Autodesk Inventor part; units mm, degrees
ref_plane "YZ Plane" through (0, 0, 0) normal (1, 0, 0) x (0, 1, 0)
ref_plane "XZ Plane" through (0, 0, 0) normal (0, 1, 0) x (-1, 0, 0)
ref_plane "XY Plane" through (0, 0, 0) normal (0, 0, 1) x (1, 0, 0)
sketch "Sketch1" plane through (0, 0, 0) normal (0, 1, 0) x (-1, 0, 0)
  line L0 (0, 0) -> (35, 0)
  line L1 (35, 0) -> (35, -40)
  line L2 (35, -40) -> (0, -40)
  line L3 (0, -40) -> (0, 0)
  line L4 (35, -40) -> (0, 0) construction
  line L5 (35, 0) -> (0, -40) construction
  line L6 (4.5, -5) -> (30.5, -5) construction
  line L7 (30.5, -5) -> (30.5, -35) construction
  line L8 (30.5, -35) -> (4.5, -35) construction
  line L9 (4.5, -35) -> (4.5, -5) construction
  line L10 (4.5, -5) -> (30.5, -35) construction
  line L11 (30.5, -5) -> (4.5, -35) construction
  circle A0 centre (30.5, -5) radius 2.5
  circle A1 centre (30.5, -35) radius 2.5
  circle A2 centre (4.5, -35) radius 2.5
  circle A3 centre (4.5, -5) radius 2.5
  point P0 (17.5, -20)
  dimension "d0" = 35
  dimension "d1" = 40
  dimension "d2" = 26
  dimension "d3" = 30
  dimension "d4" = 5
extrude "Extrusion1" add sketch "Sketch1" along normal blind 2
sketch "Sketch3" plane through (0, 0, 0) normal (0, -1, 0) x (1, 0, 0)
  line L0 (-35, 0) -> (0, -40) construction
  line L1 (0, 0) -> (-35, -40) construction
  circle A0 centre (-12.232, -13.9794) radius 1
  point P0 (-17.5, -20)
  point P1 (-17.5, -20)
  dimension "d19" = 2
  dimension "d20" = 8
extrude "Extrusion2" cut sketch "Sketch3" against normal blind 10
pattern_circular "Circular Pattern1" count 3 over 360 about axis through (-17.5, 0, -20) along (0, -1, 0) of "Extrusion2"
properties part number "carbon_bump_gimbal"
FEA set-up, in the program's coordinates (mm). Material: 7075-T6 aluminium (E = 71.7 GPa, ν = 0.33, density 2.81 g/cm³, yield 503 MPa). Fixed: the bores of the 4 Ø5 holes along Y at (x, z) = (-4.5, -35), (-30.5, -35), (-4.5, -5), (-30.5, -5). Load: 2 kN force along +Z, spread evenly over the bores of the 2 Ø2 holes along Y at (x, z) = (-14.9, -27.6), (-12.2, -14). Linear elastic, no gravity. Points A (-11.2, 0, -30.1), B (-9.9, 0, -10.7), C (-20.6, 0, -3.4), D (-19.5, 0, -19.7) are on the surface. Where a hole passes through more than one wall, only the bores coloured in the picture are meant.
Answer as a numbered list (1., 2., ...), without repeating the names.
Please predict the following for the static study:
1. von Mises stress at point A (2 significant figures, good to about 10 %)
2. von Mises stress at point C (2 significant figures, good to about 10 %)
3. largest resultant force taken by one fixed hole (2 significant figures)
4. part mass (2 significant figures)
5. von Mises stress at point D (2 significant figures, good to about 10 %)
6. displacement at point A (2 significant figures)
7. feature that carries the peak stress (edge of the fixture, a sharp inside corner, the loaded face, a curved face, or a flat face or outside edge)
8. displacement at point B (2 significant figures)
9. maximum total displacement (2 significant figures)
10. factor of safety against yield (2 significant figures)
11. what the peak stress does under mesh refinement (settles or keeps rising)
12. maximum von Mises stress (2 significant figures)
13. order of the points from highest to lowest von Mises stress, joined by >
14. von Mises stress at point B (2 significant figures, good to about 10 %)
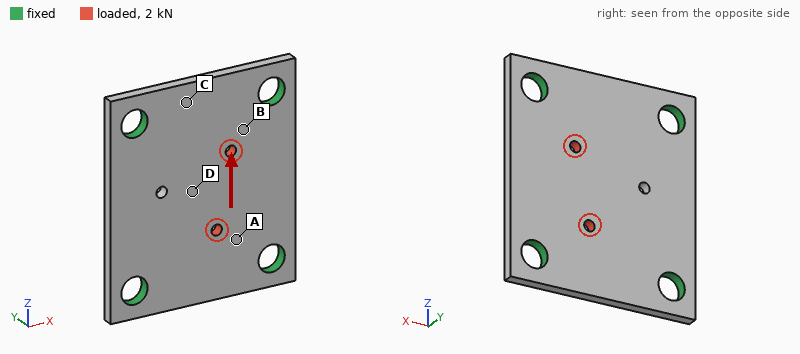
1. 36 MPa
2. 10 MPa
3. 700 N
4. 7.4 g
5. 22 MPa
6. 4.5 µm
7. the loaded face
8. 4.2 µm
9. 8.7 µm
10. 3.5
11. settles
12. 140 MPa
13. B > A > D > C
14. 47 MPa
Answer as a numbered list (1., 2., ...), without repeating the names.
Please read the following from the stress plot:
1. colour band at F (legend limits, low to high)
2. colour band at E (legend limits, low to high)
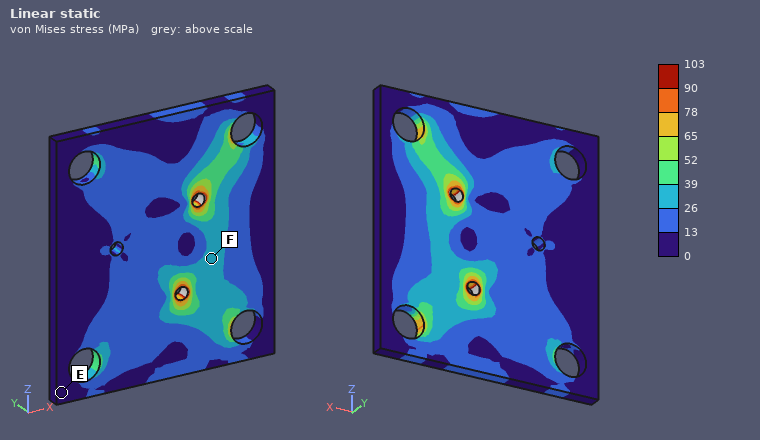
1. 26 to 39 MPa
2. 0 to 13 MPa
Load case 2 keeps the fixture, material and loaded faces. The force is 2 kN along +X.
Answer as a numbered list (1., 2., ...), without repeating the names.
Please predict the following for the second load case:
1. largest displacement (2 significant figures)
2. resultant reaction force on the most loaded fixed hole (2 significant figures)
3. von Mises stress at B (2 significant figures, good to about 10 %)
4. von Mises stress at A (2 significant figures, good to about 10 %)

1. 8.7 µm
2. 620 N
3. 40 MPa
4. 42 MPa
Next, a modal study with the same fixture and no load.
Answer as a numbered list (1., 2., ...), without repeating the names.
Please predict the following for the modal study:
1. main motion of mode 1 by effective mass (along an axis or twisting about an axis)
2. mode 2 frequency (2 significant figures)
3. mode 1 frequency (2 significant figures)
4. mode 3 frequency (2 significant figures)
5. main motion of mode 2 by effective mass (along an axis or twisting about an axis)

1. along Y
2. 16 kHz
3. 11 kHz
4. 18 kHz
5. twisting about Z
